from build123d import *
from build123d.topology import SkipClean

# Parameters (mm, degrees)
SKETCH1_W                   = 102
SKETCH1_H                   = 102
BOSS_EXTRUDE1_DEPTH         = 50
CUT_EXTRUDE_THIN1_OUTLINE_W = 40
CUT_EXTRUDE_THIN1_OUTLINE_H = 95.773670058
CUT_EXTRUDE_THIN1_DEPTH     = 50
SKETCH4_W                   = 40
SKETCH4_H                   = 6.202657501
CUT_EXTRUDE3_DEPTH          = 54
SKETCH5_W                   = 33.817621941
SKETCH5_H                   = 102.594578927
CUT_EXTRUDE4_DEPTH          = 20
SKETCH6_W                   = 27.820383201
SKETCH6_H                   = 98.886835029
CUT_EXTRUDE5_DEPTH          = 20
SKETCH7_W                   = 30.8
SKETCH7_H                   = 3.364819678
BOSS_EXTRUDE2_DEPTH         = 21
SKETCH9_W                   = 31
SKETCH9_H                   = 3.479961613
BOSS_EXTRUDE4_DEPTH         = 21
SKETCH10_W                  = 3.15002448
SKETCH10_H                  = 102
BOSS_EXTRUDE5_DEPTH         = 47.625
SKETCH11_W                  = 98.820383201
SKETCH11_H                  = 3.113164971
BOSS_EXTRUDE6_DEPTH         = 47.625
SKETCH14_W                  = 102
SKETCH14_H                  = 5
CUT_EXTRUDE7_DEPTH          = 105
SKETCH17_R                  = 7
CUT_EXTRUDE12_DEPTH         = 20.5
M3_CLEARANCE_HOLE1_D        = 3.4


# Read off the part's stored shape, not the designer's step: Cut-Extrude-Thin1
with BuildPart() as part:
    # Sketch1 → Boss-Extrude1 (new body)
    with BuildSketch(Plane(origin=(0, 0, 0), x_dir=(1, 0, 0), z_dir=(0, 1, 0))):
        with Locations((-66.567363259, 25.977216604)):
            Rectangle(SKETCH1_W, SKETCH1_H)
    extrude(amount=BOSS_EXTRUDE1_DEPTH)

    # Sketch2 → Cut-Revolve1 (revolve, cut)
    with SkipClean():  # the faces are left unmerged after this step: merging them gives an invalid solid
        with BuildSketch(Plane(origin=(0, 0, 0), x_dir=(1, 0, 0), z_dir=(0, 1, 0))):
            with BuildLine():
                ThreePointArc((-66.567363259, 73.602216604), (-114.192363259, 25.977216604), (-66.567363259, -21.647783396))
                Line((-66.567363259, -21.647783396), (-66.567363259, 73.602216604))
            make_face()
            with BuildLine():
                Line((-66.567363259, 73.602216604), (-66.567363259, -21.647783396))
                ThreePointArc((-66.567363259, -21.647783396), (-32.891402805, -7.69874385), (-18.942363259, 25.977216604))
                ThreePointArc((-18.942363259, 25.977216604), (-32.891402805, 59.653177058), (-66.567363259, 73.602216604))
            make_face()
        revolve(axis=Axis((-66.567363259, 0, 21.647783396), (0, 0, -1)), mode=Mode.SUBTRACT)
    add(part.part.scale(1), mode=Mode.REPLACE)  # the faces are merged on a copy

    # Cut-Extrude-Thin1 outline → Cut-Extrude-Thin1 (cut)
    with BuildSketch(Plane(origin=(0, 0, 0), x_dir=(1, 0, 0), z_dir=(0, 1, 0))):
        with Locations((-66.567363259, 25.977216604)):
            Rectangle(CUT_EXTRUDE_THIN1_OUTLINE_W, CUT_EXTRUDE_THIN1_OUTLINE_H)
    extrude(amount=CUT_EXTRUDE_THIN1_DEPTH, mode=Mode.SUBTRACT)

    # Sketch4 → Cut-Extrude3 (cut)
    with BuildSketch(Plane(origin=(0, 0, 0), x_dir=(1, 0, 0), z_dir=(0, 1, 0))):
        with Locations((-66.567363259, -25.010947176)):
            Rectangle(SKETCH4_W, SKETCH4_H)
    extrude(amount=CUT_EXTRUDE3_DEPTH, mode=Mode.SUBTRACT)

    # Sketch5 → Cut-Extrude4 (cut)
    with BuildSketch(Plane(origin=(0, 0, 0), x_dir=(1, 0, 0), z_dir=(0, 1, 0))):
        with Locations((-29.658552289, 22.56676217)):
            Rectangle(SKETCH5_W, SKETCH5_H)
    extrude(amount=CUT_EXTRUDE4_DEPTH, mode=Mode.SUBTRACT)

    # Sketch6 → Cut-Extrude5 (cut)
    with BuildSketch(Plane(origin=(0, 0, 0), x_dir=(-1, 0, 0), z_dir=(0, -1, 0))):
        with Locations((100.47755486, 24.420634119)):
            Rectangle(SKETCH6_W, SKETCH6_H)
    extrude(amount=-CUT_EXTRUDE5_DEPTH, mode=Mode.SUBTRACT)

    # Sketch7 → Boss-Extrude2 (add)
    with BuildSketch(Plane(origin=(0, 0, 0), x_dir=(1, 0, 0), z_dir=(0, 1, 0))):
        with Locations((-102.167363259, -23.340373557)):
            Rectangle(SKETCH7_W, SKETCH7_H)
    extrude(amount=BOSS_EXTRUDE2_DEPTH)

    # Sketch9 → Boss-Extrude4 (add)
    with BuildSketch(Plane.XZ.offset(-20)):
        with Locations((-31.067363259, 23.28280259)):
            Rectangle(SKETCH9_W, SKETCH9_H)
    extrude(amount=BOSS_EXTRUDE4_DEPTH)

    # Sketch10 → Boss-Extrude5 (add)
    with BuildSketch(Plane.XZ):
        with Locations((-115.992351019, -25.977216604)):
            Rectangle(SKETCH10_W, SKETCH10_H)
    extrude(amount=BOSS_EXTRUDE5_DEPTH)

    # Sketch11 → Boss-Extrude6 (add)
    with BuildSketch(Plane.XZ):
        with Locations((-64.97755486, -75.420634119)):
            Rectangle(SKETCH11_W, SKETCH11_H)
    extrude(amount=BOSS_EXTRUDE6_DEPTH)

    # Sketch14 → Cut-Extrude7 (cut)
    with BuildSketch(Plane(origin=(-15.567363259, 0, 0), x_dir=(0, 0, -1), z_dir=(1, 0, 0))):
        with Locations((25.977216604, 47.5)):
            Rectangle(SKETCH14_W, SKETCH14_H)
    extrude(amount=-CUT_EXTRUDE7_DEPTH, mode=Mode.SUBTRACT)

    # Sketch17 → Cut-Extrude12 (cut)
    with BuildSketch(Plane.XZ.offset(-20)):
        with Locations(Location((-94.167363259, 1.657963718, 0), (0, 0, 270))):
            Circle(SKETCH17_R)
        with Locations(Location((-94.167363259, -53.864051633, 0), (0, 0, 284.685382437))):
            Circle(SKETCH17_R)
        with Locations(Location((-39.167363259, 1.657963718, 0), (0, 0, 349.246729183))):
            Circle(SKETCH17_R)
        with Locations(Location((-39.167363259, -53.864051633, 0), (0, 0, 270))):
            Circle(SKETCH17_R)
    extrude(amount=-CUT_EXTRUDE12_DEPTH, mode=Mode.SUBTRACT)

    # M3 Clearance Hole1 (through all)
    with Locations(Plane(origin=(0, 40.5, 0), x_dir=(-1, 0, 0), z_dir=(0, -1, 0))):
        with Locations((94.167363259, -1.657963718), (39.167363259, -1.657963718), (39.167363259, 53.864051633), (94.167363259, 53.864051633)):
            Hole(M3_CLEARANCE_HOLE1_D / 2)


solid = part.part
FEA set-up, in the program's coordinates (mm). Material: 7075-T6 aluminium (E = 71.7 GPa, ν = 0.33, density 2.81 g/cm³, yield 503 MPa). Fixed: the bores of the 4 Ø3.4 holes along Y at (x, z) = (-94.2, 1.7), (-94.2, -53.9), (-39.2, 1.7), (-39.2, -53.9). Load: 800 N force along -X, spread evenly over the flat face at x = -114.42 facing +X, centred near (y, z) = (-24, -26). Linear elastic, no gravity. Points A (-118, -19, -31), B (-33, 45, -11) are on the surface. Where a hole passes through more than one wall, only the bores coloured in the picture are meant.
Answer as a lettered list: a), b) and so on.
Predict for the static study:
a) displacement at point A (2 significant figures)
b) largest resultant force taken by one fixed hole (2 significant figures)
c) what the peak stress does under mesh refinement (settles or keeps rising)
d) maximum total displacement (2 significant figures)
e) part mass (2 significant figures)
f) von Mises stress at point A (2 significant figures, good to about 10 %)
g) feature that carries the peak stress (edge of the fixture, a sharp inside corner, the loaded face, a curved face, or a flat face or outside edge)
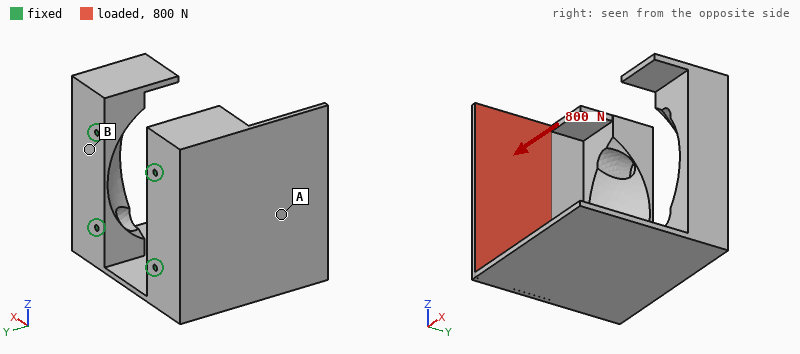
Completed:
a) 0.77 mm
b) 950 N
c) keeps rising
d) 1.7 mm
e) 480 g
f) 41 MPa
g) a sharp inside corner
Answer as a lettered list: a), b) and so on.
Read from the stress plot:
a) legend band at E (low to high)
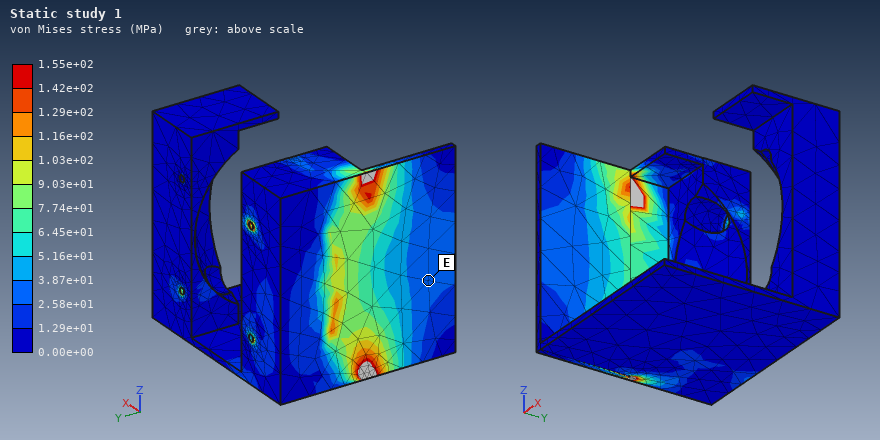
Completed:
a) 2.58e+01 to 3.87e+01 MPa
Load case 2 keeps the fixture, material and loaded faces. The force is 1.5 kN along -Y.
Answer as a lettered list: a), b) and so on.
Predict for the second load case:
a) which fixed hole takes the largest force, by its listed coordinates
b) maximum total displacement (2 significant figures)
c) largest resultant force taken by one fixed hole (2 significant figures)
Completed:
a) (-94.2, -53.9)
b) 93 µm
c) 1.2 kN
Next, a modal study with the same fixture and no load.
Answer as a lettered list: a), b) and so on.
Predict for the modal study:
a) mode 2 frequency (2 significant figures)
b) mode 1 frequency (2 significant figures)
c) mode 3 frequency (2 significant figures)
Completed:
a) 670 Hz
b) 570 Hz
c) 1200 Hz
